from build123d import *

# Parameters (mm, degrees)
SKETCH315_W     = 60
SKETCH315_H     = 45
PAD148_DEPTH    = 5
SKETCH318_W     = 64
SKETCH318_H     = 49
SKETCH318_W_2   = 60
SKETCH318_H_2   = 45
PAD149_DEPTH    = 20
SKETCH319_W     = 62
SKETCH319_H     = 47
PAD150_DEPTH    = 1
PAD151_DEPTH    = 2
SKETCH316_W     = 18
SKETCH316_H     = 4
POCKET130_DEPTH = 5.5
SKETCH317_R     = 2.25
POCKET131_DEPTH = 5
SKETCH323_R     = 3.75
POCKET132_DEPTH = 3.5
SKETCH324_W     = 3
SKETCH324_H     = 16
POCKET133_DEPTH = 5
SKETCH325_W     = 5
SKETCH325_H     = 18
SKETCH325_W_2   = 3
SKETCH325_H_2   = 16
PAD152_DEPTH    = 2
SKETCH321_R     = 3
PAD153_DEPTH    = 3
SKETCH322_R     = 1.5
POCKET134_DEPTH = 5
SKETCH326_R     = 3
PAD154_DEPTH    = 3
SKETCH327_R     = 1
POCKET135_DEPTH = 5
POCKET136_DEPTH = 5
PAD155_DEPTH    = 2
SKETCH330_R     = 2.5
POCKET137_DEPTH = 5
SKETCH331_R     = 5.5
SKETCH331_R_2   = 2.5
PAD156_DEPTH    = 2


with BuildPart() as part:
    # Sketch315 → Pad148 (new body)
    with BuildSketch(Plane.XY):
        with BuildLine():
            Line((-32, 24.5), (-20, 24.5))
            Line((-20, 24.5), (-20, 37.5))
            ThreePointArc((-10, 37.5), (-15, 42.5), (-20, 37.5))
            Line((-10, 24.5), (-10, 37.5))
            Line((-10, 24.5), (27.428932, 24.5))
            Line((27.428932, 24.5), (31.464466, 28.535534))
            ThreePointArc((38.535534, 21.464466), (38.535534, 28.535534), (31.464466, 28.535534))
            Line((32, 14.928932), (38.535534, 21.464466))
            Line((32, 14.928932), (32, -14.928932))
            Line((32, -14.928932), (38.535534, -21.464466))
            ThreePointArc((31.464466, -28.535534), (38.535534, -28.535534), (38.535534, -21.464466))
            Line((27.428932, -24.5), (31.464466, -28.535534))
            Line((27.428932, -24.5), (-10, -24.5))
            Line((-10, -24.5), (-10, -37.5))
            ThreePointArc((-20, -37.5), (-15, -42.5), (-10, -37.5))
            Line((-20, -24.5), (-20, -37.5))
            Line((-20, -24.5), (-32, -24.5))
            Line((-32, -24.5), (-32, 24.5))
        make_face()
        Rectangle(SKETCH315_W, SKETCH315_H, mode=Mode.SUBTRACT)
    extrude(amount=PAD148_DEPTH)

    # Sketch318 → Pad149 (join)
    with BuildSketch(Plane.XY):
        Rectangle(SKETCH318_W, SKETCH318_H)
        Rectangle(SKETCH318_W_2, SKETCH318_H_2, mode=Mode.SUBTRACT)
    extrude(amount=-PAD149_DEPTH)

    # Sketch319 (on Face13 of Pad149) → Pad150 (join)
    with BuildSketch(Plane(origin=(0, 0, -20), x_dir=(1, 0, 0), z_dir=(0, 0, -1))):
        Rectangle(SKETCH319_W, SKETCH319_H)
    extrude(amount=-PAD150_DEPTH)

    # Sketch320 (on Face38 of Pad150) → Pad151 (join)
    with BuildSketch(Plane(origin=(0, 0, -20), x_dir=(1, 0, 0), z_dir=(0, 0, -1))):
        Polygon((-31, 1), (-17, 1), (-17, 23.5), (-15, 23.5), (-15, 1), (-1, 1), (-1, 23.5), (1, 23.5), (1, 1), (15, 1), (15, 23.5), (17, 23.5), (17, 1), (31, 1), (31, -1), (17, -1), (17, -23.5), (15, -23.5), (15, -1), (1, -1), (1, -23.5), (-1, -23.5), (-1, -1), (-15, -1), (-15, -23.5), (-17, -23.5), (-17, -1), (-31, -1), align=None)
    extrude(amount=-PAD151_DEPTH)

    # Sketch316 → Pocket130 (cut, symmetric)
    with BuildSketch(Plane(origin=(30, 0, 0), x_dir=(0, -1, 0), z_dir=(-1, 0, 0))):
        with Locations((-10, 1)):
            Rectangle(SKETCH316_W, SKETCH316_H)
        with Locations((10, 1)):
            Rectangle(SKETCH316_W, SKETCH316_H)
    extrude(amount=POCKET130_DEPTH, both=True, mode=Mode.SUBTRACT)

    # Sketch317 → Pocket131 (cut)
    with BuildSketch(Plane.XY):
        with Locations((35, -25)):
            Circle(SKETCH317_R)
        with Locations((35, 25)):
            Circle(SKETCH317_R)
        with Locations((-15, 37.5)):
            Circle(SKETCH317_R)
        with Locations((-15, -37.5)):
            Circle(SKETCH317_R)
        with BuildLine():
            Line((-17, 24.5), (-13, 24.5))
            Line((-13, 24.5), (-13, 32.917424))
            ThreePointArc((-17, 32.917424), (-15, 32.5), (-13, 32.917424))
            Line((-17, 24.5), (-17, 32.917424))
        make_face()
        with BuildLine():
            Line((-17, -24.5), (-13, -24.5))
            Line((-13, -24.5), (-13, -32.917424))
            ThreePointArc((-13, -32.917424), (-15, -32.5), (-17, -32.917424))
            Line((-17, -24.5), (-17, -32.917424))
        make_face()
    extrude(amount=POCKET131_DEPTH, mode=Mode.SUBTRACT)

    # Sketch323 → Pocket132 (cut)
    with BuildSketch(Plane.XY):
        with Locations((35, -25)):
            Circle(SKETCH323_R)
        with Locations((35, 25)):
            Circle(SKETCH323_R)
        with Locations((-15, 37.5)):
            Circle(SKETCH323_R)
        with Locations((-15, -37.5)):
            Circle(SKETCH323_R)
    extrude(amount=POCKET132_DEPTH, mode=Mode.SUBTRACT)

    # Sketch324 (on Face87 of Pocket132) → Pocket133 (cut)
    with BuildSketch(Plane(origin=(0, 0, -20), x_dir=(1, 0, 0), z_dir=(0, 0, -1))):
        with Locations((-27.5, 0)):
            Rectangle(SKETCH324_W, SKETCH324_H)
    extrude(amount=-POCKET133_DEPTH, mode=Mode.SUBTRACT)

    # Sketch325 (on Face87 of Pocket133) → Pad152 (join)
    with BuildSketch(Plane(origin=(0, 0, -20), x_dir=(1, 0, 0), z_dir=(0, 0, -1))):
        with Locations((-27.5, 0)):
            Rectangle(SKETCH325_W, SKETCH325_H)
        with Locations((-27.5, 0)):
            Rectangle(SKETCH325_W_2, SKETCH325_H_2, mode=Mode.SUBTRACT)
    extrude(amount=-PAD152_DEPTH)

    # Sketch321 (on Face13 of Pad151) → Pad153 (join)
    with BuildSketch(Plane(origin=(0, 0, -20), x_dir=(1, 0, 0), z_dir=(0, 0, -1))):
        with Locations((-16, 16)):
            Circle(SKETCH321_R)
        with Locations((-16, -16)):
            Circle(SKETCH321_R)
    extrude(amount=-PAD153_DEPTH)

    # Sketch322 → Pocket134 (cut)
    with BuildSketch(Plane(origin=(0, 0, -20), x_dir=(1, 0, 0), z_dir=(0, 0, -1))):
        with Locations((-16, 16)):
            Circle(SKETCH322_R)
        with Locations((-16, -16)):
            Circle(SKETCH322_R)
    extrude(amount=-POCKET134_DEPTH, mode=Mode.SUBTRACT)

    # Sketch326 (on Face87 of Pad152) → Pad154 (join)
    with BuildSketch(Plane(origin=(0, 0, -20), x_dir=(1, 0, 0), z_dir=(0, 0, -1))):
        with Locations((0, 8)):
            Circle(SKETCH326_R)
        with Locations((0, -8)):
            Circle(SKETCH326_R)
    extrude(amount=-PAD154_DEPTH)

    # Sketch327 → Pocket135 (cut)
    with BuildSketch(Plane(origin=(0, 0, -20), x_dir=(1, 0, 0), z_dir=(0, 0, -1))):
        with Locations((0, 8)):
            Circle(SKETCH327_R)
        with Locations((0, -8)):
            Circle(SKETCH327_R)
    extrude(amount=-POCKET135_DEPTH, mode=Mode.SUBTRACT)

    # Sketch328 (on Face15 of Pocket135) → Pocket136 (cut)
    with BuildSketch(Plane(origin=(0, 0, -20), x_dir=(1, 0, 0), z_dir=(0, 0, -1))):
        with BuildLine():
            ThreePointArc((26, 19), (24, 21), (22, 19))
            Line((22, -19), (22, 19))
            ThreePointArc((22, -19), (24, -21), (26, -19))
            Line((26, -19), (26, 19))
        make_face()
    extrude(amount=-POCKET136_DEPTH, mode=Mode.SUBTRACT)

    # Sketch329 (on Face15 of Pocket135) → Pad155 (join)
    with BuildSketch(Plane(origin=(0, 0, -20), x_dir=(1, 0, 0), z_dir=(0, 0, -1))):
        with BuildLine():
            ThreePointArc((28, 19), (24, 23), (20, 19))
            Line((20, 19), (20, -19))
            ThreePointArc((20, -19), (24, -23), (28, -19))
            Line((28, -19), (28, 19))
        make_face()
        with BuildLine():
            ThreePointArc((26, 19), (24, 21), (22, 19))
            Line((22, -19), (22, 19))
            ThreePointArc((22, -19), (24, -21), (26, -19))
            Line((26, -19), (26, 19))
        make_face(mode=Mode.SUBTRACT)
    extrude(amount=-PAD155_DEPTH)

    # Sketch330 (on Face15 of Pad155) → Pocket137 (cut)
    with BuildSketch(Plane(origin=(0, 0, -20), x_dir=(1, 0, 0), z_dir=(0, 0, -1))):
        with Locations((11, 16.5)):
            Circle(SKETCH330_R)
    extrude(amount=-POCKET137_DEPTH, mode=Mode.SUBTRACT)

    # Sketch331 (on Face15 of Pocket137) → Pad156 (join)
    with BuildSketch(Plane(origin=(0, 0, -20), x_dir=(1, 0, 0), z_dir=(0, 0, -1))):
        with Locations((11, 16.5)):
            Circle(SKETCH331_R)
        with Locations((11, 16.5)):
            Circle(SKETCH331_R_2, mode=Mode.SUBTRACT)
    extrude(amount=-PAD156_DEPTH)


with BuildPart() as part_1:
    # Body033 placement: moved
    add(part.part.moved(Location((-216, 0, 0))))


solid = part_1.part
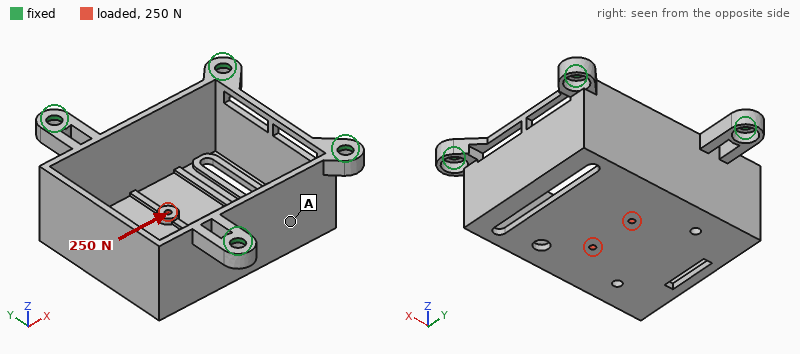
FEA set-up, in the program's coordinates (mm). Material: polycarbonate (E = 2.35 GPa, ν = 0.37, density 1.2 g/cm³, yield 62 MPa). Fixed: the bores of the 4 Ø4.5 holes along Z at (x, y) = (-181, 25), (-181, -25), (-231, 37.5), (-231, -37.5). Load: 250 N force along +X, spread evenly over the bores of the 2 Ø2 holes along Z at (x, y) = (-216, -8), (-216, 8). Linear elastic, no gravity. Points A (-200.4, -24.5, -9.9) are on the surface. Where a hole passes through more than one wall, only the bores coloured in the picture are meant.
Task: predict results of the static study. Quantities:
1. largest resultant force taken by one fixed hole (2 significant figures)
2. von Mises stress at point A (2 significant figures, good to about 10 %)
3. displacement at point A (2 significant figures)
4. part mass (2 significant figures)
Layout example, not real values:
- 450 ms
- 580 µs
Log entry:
- 120 N
- 2.6 MPa
- 0.23 mm
- 18 g
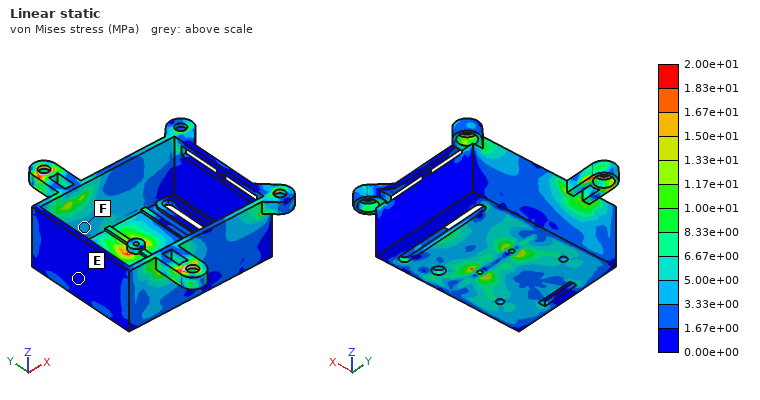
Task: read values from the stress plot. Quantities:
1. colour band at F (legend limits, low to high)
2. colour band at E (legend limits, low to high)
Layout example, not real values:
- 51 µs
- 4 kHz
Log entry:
- 3.33e+00 to 5.00e+00 MPa
- 0.00e+00 to 1.67e+00 MPa
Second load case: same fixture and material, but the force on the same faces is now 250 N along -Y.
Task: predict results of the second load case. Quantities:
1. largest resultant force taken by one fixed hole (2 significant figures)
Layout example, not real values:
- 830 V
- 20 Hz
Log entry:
- 110 N
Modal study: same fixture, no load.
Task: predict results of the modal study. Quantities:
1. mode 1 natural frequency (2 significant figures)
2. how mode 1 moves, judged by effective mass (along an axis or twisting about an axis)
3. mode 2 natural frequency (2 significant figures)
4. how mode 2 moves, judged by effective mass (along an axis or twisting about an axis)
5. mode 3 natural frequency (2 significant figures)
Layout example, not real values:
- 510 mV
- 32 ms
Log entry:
- 710 Hz
- along Z
- 850 Hz
- along Y
- 990 Hz
